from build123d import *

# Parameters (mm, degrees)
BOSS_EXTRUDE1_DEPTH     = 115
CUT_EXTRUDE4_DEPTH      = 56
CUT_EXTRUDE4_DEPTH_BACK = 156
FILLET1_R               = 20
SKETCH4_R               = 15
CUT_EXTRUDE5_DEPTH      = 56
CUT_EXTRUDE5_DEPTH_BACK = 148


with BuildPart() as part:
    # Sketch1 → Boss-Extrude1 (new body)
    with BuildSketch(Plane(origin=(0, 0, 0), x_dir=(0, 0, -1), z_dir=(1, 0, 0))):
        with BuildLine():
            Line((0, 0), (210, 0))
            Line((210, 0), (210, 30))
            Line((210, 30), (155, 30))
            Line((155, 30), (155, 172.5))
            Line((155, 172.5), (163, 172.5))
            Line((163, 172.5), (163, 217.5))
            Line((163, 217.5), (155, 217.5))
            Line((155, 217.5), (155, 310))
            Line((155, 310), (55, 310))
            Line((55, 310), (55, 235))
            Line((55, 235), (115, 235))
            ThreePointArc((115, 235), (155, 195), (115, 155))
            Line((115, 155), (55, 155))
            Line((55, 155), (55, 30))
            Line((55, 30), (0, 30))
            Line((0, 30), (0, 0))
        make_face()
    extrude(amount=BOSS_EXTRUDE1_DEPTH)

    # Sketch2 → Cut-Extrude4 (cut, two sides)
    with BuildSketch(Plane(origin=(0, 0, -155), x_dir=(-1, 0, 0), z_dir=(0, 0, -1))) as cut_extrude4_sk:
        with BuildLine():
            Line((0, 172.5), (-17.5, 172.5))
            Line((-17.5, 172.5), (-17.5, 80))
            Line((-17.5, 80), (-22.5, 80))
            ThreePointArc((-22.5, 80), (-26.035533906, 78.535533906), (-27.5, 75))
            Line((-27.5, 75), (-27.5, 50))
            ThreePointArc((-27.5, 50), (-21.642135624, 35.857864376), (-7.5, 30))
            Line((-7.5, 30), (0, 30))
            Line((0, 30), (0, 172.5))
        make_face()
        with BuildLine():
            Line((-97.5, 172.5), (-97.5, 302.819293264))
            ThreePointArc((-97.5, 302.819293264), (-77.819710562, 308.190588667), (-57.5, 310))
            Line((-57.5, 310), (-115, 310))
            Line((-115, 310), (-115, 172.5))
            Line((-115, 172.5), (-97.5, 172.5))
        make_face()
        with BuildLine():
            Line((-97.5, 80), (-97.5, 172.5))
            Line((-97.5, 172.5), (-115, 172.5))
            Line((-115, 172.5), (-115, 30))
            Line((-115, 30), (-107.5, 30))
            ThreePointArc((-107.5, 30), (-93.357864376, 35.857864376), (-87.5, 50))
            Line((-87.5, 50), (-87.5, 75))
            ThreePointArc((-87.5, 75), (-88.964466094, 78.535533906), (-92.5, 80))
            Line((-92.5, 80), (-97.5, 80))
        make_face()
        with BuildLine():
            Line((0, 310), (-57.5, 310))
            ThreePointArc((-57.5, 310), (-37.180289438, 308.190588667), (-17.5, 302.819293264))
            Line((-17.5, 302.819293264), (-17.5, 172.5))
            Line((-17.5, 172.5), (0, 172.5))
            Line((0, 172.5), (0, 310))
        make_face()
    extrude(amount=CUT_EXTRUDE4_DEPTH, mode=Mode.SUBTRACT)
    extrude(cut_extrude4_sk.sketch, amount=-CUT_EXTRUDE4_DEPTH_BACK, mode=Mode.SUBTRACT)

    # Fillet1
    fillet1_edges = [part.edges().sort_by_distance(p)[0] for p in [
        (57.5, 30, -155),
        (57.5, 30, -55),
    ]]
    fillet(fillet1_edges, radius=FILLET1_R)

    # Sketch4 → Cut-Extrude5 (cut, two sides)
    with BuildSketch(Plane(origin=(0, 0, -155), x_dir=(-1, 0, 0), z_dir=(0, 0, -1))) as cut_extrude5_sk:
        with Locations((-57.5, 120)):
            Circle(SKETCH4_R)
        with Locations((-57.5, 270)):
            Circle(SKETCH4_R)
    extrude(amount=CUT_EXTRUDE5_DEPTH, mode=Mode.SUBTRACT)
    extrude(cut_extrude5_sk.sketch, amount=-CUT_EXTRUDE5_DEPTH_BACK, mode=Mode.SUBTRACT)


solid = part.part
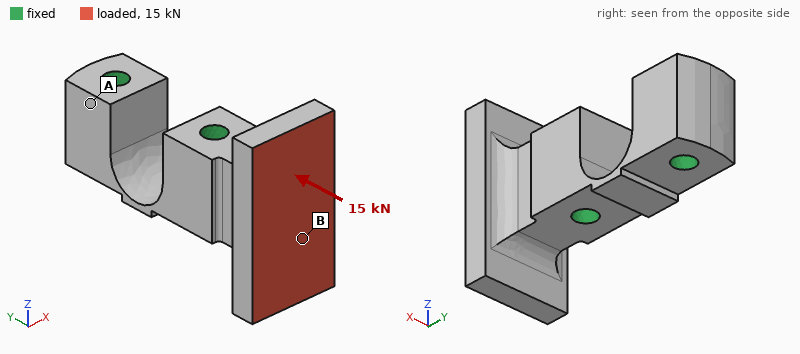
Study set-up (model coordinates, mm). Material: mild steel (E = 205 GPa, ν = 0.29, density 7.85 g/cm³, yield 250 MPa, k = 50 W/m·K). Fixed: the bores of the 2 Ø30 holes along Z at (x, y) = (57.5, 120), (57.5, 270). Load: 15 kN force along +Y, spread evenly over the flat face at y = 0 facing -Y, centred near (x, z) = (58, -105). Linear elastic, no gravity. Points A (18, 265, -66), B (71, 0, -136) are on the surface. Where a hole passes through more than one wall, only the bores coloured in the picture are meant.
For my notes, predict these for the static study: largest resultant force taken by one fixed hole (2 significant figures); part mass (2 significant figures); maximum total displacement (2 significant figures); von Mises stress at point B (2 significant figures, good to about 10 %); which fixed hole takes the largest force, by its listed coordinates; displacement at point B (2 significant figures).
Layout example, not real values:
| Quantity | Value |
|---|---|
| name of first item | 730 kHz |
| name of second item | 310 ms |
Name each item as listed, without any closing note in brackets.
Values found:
| Quantity | Value |
|---|---|
| largest resultant force taken by one fixed hole | 15 kN |
| part mass | 17 kg |
| maximum total displacement | 5.2 µm |
| von Mises stress at point B | 3.9 MPa |
| which fixed hole takes the largest force, by its listed coordinates | (57.5, 120) |
| displacement at point B | 1.1 µm |
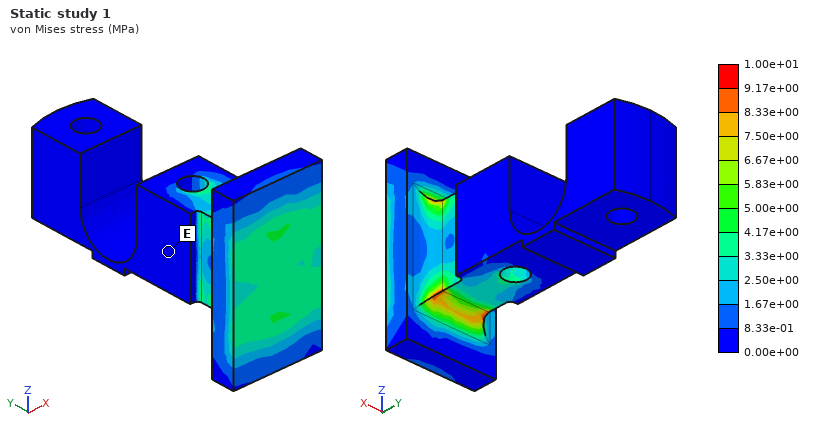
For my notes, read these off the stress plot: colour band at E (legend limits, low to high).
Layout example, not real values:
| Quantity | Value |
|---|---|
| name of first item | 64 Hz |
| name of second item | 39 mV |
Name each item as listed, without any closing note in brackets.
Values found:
| Quantity | Value |
|---|---|
| colour band at E | 0.00e+00 to 8.33e-01 MPa |
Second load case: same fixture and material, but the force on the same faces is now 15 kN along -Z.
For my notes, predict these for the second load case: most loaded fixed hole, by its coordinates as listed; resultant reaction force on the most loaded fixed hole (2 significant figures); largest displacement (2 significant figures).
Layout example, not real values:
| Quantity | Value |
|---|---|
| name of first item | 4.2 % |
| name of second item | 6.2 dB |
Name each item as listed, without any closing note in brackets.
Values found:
| Quantity | Value |
|---|---|
| most loaded fixed hole, by its coordinates as listed | (57.5, 120) |
| resultant reaction force on the most loaded fixed hole | 15 kN |
| largest displacement | 16 µm |
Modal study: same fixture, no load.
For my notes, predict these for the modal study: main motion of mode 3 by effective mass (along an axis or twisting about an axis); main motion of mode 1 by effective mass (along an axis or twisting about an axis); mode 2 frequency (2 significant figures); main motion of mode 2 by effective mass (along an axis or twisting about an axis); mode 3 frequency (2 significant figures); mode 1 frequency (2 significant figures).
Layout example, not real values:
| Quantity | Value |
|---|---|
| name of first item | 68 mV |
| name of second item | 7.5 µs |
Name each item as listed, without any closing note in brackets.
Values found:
| Quantity | Value |
|---|---|
| main motion of mode 3 by effective mass | along Z |
| main motion of mode 1 by effective mass | along X |
| mode 2 frequency | 2200 Hz |
| main motion of mode 2 by effective mass | twisting about Y |
| mode 3 frequency | 2300 Hz |
| mode 1 frequency | 1800 Hz |
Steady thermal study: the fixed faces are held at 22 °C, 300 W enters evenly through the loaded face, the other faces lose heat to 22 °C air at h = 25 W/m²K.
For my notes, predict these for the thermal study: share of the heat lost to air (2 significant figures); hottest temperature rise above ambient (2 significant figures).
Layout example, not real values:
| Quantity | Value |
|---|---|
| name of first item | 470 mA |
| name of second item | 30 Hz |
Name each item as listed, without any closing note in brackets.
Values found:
| Quantity | Value |
|---|---|
| share of the heat lost to air | 27 % |
| hottest temperature rise above ambient | 76 K |
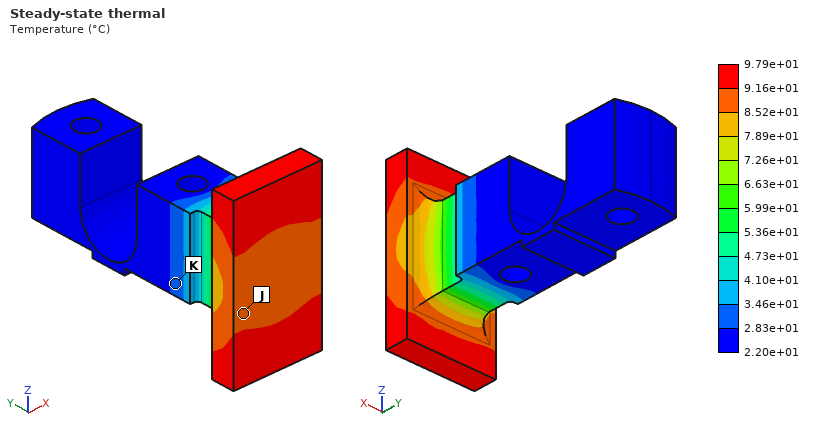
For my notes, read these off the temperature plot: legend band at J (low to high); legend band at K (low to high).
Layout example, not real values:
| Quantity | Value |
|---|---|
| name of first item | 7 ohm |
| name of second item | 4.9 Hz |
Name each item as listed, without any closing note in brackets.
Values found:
| Quantity | Value |
|---|---|
| legend band at J | 8.52e+01 to 9.16e+01 °C |
| legend band at K | 2.83e+01 to 3.46e+01 °C |
